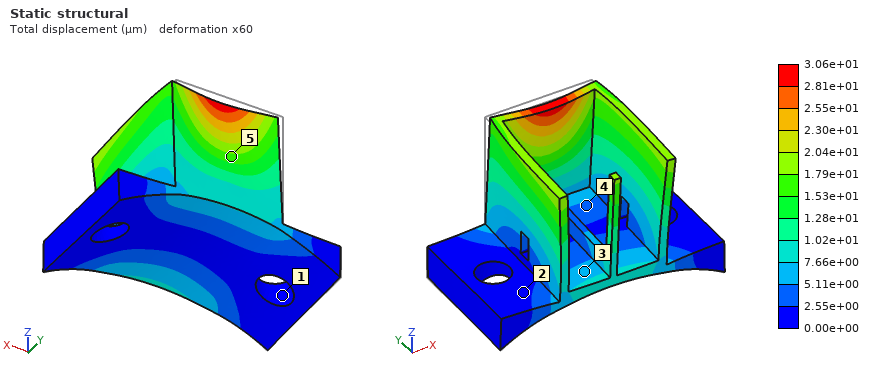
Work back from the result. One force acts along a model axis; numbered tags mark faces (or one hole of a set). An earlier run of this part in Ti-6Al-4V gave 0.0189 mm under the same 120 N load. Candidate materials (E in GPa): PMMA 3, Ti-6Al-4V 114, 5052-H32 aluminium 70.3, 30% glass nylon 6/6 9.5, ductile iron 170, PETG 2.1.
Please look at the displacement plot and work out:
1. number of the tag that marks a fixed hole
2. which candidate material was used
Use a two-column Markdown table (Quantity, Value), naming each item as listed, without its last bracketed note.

| Quantity | Value |
|---|---|
| number of the tag that marks a fixed hole | 1 |
| which candidate material was used | 5052-H32 aluminium |
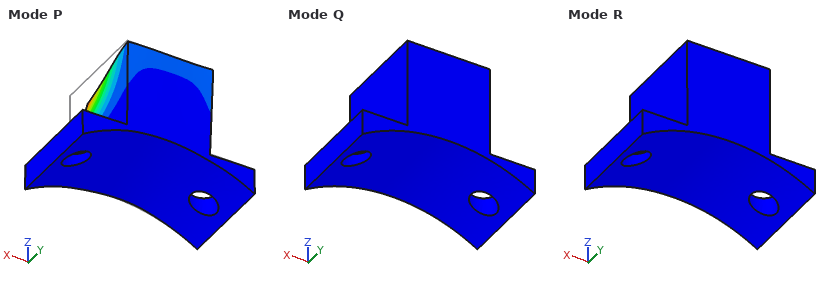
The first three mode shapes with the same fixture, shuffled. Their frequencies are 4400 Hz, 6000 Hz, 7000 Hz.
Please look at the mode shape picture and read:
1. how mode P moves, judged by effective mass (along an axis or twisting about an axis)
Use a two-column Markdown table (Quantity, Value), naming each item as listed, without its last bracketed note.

| Quantity | Value |
|---|---|
| how mode P moves, judged by effective mass | along X |
